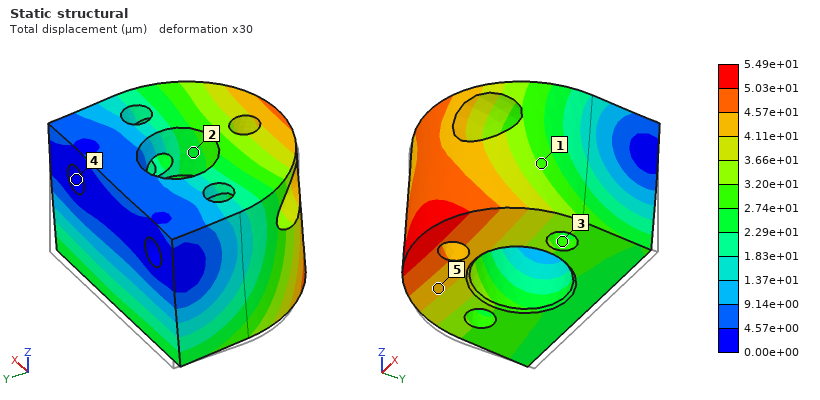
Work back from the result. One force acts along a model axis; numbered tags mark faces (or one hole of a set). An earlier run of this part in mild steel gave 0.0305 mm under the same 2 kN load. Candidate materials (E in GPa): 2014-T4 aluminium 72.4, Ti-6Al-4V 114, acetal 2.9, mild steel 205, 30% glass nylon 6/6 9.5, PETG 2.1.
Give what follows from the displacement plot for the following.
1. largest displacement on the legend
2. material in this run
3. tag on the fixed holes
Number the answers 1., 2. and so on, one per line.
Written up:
1. 5.49e+01 µm
2. Ti-6Al-4V
3. 4
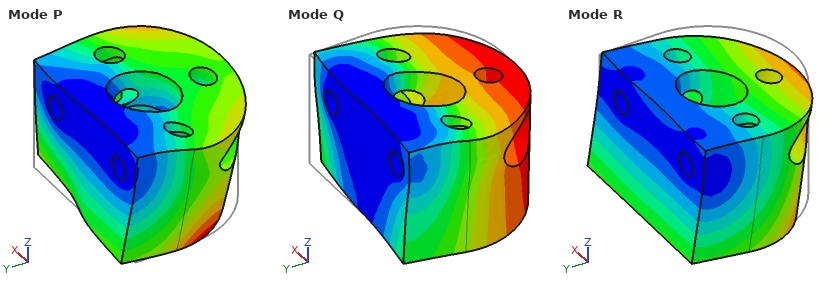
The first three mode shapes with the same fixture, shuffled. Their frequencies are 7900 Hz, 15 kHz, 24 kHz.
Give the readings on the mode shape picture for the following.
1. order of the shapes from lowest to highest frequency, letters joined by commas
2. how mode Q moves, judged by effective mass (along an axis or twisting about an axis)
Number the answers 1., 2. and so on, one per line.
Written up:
1. R, Q, P
2. along X
